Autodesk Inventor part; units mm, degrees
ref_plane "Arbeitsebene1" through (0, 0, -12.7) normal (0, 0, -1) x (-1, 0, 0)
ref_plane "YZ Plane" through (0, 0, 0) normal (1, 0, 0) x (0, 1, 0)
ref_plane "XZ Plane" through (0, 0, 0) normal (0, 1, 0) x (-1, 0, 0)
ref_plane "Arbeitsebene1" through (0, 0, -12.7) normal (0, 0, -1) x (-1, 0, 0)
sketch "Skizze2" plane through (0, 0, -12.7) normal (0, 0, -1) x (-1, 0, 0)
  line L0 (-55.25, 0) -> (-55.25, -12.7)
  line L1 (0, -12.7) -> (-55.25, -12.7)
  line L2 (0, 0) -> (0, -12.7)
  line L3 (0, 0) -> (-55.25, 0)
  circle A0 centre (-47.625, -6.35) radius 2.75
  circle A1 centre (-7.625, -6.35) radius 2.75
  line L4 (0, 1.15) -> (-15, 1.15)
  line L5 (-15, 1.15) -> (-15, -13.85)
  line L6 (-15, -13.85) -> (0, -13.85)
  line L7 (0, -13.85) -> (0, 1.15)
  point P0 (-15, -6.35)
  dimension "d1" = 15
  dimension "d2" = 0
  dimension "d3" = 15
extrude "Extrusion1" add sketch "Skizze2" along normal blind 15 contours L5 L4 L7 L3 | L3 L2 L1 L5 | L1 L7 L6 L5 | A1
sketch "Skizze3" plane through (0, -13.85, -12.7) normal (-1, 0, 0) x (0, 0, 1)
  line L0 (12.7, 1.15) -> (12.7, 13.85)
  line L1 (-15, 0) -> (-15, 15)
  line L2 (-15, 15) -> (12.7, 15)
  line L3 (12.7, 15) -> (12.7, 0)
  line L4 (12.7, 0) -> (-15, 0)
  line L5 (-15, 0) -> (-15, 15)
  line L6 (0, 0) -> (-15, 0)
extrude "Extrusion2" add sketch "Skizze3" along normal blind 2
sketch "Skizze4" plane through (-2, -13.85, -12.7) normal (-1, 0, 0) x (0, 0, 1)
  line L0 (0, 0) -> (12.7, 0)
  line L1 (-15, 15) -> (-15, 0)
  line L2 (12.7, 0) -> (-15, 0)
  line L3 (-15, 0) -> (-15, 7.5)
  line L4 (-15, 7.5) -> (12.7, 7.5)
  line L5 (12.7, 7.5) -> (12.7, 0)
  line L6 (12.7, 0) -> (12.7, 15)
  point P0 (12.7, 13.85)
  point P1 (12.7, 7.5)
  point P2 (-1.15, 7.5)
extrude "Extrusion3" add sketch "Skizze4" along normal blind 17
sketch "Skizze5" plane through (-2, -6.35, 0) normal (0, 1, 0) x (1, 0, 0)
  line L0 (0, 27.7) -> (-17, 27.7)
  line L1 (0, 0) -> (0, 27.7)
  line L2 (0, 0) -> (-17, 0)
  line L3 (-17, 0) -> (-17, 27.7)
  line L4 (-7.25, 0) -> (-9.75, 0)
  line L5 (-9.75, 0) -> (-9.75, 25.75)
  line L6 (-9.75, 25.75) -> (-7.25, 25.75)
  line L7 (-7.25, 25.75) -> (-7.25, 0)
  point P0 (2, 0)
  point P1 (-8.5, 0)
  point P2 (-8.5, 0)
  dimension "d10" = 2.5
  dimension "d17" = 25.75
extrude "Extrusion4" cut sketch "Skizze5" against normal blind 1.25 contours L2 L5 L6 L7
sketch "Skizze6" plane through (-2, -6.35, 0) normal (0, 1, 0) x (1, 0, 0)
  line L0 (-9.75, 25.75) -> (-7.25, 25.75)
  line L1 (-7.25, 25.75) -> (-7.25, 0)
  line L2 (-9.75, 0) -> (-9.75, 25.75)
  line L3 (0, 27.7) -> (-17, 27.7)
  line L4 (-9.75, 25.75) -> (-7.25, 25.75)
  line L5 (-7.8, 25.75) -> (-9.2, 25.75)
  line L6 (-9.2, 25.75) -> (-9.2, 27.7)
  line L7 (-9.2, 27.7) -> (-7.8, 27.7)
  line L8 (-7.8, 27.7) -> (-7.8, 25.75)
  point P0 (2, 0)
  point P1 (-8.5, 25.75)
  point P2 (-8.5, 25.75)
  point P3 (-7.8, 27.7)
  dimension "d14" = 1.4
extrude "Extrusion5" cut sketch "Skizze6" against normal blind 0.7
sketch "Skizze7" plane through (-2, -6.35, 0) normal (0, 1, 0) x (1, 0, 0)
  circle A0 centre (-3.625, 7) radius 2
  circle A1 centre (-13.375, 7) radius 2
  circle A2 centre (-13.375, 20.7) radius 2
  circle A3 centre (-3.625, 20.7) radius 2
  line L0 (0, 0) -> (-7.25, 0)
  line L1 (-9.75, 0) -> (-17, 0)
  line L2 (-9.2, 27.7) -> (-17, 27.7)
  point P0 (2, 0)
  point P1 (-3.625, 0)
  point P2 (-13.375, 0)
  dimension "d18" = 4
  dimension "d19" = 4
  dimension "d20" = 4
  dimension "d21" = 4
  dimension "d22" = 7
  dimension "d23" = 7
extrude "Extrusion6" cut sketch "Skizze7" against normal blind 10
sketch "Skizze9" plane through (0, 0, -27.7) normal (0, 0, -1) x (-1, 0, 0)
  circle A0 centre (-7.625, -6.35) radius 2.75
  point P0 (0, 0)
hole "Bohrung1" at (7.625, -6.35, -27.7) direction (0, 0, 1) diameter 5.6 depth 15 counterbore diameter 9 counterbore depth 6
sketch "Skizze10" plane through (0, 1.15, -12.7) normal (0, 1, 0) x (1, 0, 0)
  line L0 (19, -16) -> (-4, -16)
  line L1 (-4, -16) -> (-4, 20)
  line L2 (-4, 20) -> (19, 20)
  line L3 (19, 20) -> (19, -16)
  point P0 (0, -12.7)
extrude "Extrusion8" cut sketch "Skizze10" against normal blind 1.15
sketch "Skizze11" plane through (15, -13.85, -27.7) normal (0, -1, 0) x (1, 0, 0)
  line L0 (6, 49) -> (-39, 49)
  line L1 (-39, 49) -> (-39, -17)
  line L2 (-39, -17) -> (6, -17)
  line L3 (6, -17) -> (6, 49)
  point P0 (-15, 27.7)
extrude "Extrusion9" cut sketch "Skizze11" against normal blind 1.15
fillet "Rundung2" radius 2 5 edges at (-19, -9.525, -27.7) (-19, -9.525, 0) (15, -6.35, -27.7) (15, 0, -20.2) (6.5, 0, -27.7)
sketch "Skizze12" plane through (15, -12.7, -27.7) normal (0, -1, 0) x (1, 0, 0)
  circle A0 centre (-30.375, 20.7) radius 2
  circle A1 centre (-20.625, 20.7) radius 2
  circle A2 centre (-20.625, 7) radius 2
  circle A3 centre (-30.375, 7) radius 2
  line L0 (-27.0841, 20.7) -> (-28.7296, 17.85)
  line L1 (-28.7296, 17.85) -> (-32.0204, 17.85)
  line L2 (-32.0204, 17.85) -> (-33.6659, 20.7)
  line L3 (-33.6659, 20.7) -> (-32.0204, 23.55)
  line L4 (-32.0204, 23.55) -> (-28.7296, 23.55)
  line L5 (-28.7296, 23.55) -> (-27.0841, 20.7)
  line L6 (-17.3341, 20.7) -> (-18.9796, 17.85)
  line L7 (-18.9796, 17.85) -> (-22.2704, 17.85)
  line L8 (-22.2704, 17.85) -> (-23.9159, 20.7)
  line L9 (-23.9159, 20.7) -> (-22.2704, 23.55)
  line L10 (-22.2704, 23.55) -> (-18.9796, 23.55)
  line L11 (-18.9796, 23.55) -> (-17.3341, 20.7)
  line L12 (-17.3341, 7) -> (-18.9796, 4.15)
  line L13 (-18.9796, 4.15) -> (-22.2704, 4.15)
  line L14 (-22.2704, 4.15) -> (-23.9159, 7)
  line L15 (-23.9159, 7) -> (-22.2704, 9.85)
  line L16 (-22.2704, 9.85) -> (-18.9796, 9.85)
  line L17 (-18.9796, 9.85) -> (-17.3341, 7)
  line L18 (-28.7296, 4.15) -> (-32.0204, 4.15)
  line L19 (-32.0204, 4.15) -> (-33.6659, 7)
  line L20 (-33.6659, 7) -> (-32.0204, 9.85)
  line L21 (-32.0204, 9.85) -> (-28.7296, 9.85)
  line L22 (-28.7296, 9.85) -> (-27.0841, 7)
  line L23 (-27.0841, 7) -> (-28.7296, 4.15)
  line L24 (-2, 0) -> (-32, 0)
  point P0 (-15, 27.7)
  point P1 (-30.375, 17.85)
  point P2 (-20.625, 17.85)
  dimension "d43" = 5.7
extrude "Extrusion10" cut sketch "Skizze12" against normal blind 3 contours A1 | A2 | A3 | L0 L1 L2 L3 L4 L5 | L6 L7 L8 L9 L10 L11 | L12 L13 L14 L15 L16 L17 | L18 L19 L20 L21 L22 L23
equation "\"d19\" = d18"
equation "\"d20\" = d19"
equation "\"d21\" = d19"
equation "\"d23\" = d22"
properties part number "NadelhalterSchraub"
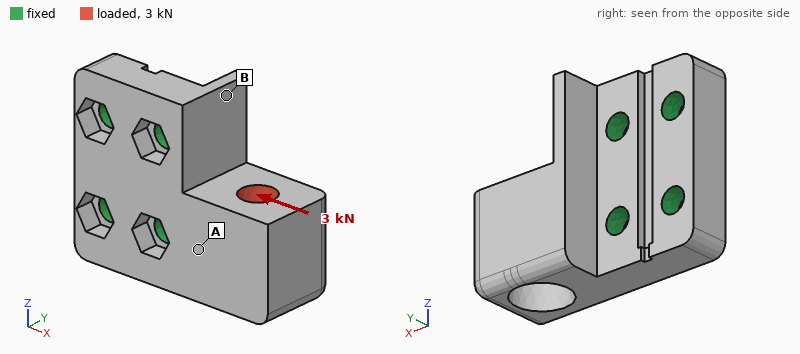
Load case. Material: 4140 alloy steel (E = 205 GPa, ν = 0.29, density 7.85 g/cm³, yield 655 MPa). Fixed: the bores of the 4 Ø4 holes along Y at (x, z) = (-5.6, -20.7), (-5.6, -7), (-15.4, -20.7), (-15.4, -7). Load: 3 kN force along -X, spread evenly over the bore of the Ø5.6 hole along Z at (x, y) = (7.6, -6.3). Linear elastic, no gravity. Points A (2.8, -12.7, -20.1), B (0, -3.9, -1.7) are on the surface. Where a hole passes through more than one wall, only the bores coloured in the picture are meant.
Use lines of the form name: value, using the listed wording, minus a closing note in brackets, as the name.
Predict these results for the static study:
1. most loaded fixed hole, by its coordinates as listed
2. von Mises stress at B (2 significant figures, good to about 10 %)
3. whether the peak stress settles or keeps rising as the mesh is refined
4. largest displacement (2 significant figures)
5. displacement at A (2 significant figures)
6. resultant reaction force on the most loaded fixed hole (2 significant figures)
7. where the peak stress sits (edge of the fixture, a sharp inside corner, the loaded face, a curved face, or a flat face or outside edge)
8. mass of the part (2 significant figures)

most loaded fixed hole, by its coordinates as listed: (-5.6, -20.7)
von Mises stress at B: 23 MPa
whether the peak stress settles or keeps rising as the mesh is refined: keeps rising
largest displacement: 20 µm
displacement at A: 5.0 µm
resultant reaction force on the most loaded fixed hole: 2.2 kN
where the peak stress sits: edge of the fixture
mass of the part: 42 g
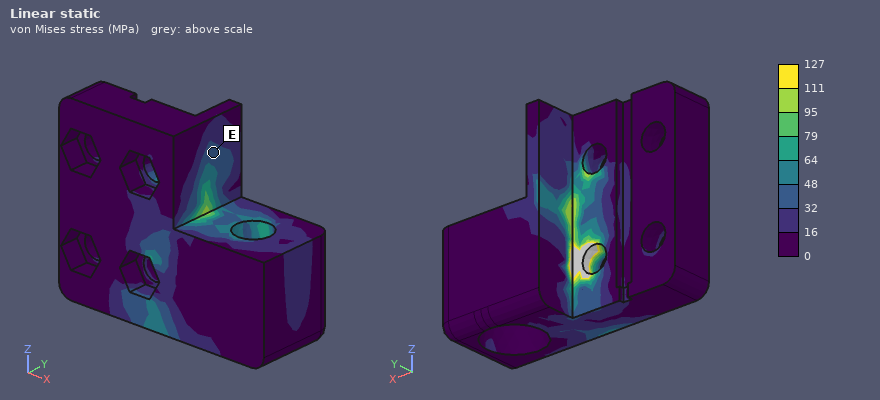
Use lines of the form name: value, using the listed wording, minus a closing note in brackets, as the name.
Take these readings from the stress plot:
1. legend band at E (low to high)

legend band at E: 32 to 48 MPa
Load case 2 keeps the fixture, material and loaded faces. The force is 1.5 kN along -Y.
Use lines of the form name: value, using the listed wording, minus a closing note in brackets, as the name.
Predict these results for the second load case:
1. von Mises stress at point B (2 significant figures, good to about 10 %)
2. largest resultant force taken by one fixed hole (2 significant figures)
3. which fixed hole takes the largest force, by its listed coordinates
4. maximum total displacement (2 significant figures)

von Mises stress at point B: 31 MPa
largest resultant force taken by one fixed hole: 2.0 kN
which fixed hole takes the largest force, by its listed coordinates: (-5.6, -20.7)
maximum total displacement: 43 µm
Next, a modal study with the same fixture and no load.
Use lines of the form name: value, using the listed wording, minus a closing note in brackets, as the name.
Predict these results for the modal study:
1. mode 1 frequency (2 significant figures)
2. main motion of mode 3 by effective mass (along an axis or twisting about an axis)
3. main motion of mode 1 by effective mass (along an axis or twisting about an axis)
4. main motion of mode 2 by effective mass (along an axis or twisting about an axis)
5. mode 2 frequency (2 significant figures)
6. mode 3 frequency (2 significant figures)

mode 1 frequency: 8100 Hz
main motion of mode 3 by effective mass: twisting about X
main motion of mode 1 by effective mass: along Y
main motion of mode 2 by effective mass: along Z
mode 2 frequency: 17 kHz
mode 3 frequency: 26 kHz
